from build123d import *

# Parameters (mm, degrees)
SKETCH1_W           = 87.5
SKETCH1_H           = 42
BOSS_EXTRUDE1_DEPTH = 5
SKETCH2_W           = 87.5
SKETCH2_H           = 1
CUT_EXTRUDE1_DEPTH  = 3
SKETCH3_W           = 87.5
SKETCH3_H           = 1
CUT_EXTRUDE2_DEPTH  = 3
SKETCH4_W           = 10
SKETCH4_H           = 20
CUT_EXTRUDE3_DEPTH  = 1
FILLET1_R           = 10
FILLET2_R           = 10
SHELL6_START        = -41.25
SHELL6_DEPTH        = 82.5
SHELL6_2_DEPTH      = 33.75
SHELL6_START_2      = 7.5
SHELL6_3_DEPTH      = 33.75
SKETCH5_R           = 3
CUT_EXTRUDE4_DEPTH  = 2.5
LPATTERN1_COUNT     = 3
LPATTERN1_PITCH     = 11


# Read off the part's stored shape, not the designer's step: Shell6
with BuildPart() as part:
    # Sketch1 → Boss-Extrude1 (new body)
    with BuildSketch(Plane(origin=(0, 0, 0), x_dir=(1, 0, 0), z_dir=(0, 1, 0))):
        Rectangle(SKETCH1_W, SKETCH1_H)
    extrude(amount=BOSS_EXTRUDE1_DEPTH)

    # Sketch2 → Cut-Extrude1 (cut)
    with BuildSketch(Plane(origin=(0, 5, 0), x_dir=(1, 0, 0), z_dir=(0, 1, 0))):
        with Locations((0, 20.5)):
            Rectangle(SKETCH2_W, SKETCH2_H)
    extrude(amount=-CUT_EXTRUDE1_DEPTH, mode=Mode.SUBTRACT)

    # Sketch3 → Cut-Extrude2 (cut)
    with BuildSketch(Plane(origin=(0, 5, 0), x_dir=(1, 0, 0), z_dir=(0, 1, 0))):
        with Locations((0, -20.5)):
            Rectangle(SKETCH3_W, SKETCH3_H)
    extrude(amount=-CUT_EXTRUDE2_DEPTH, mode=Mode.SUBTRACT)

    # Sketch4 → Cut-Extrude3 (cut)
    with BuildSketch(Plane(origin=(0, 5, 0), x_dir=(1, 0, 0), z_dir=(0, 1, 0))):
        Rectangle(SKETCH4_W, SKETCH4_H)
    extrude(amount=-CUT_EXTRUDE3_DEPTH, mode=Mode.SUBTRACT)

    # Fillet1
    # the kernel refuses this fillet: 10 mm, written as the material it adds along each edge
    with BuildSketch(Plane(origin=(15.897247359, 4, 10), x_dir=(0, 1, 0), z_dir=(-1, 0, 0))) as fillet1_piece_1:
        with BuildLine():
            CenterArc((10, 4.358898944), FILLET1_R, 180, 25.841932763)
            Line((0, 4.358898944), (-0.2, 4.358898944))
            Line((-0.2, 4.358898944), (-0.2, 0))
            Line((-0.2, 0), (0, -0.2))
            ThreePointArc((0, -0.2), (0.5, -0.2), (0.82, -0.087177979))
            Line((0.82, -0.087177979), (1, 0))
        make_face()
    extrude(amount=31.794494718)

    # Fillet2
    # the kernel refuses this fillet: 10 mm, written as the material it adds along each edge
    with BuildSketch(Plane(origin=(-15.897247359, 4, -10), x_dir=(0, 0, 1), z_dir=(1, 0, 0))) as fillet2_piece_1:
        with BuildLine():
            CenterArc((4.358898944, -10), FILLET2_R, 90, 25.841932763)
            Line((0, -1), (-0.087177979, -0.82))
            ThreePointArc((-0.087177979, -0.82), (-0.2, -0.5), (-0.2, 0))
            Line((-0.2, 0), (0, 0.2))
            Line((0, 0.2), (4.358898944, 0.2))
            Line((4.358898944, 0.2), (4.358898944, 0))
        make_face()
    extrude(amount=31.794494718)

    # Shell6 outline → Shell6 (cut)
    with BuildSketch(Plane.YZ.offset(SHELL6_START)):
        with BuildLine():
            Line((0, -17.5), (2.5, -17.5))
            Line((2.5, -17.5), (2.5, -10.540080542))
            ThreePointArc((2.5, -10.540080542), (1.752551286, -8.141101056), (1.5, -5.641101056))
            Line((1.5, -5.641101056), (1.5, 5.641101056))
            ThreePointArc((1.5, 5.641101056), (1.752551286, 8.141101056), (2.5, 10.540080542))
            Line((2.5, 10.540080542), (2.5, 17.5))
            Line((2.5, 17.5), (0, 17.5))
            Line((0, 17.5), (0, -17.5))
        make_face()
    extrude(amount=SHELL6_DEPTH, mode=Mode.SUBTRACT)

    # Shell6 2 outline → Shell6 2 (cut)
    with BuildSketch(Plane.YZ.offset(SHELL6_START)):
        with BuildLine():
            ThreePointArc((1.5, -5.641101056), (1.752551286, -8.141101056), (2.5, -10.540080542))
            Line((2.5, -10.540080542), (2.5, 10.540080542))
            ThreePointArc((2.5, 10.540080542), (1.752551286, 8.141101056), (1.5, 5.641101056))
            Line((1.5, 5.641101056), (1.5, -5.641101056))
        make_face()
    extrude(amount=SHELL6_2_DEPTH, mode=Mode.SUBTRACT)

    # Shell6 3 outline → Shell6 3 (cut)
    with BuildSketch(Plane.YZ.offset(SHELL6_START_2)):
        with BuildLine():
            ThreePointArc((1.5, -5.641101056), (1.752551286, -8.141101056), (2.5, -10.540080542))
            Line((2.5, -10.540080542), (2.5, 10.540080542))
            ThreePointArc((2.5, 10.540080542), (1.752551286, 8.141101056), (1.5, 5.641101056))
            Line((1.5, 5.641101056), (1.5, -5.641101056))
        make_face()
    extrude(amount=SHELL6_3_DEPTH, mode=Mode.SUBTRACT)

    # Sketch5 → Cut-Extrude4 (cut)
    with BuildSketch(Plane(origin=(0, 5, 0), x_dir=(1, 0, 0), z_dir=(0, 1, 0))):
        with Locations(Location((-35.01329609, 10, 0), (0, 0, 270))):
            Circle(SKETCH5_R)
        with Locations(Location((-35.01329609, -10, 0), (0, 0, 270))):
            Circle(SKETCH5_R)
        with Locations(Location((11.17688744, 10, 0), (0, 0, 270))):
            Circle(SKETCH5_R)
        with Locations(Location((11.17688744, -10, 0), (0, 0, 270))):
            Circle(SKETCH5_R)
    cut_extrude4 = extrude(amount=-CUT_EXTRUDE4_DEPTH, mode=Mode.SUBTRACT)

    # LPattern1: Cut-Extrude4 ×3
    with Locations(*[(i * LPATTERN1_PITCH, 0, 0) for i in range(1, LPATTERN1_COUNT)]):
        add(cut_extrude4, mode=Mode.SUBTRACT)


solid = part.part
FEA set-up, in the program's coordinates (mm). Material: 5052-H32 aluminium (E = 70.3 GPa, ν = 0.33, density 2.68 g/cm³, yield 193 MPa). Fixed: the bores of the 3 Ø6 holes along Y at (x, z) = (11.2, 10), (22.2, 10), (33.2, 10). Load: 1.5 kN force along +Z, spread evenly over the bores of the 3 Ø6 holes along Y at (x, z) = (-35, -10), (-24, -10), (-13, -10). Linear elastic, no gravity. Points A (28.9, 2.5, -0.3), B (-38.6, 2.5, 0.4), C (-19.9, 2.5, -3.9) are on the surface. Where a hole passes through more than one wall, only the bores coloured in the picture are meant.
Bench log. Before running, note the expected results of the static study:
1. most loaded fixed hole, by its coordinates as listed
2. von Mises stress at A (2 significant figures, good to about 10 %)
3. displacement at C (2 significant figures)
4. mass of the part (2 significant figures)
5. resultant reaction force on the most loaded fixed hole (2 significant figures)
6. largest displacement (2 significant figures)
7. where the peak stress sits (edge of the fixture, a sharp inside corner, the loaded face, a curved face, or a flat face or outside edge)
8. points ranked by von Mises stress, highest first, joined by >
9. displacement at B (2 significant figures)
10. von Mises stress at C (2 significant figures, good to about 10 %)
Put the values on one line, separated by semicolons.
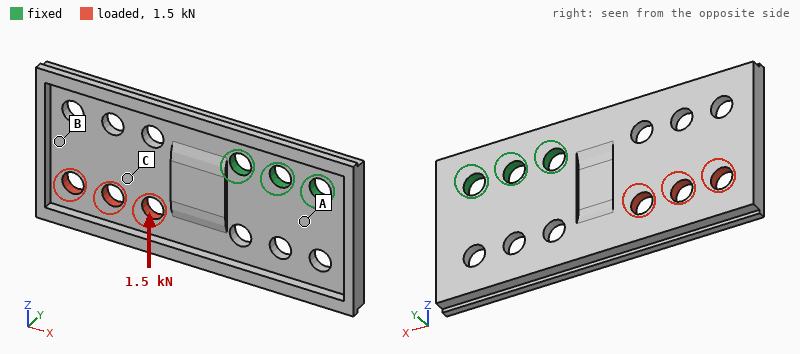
(11.2, 10); 51 MPa; 0.096 mm; 26 g; 3.2 kN; 0.17 mm; edge of the fixture; A > C > B; 0.14 mm; 25 MPa
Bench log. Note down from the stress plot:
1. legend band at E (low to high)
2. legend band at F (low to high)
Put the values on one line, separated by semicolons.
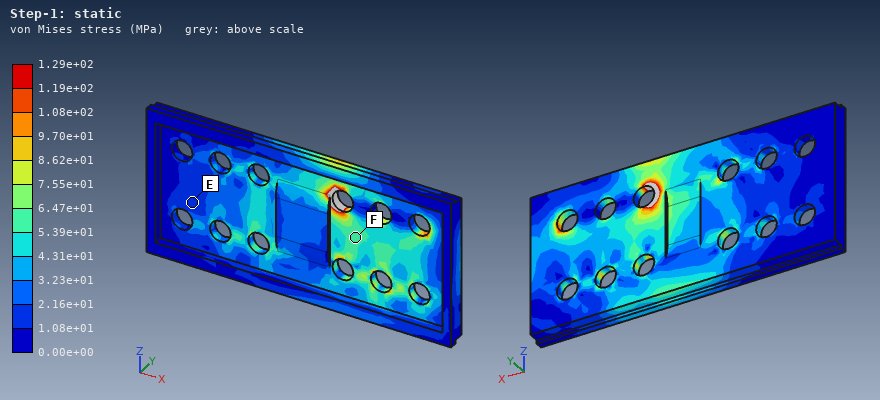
1.08e+01 to 2.16e+01 MPa; 5.39e+01 to 6.47e+01 MPa
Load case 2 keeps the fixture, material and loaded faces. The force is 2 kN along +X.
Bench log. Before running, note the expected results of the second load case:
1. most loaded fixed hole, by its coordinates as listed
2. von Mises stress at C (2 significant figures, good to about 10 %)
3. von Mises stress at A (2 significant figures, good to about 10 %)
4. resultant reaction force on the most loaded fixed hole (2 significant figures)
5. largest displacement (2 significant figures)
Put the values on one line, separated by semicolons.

(11.2, 10); 20 MPa; 42 MPa; 1.7 kN; 0.17 mm
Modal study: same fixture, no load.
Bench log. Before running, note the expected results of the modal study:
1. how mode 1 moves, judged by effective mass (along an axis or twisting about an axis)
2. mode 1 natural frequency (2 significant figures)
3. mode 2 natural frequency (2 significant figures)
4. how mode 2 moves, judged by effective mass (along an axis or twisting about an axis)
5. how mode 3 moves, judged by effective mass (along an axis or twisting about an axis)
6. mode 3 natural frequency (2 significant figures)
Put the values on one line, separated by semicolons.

along Y; 830 Hz; 1700 Hz; twisting about X; along Y; 2900 Hz
